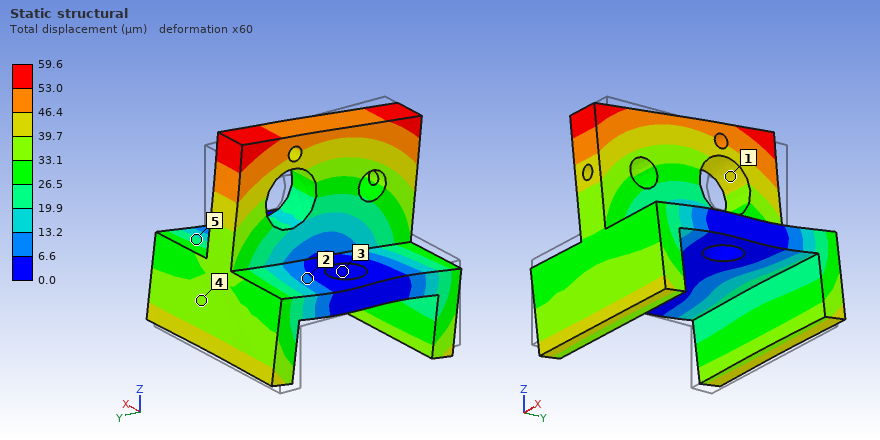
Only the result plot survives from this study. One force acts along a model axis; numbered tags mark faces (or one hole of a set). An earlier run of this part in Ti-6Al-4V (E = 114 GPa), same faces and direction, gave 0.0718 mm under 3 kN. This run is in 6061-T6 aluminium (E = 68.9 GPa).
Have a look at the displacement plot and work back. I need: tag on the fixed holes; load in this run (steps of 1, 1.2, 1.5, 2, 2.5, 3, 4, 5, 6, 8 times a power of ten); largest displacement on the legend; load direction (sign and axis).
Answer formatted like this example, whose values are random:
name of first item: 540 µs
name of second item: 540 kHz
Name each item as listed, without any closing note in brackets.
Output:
tag on the fixed holes: 3
load in this run: 1.5 kN
largest displacement on the legend: 59.6 µm
load direction: -Y
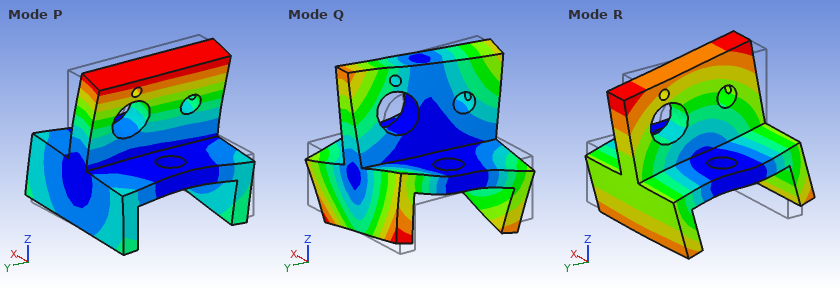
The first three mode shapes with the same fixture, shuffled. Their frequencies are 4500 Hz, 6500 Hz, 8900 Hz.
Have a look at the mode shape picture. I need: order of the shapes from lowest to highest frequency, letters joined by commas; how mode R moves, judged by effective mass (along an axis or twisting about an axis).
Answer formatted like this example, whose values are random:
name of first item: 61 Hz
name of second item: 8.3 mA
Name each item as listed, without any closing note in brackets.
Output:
order of the shapes from lowest to highest frequency, letters joined by commas: R, P, Q
how mode R moves, judged by effective mass: twisting about X
